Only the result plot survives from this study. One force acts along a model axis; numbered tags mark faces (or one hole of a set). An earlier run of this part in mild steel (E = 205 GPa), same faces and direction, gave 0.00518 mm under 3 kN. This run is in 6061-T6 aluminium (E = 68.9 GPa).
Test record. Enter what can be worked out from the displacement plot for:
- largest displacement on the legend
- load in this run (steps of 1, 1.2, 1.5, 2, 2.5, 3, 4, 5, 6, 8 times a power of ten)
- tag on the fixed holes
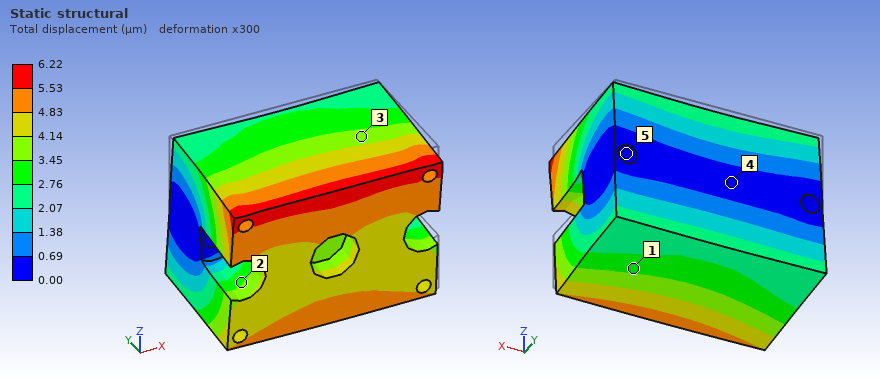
6.22 µm
1.2 kN
5
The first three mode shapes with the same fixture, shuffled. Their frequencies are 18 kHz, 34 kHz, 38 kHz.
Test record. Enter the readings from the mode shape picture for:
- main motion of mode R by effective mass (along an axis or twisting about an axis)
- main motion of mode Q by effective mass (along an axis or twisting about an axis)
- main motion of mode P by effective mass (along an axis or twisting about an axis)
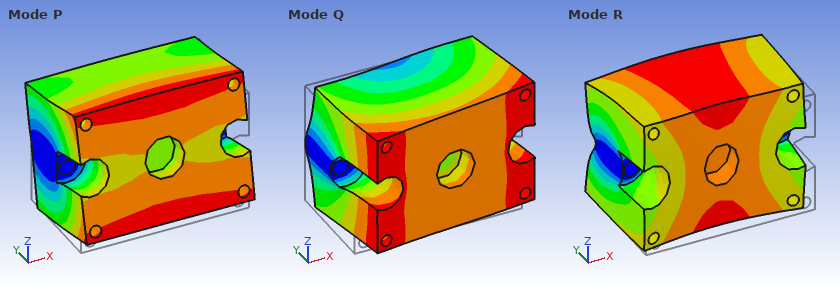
along Y
along X
along Z
